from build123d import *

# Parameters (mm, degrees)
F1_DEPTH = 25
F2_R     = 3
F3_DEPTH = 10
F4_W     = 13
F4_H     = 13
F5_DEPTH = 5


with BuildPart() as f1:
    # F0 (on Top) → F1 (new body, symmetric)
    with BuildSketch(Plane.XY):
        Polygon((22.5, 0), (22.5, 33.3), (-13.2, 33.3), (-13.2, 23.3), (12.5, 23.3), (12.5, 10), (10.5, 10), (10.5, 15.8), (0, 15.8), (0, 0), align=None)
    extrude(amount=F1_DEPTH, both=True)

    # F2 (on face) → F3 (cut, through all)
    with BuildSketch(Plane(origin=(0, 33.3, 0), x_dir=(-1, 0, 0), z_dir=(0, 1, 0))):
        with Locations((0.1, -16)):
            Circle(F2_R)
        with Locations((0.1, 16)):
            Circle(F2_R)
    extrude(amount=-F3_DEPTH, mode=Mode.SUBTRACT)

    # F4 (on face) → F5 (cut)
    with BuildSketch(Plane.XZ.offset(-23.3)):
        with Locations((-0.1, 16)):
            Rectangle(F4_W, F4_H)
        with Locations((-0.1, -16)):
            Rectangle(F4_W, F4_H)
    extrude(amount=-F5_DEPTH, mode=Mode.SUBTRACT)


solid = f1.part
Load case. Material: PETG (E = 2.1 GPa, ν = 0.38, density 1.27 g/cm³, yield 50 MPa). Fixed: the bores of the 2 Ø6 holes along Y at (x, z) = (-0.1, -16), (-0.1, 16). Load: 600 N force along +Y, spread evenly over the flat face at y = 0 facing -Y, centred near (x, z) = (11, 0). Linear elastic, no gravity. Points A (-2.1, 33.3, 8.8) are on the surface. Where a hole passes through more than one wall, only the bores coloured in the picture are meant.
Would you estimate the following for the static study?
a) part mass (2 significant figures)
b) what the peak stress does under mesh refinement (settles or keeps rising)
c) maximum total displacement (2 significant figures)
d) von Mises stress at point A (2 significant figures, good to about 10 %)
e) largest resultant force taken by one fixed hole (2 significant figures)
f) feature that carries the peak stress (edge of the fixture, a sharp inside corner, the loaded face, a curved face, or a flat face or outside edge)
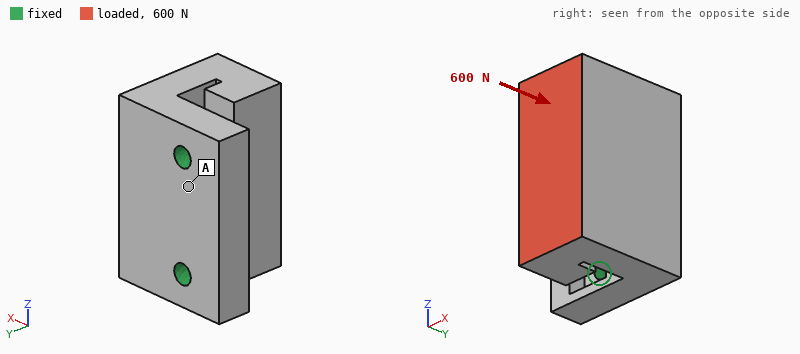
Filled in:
47 g
keeps rising
0.51 mm
3.8 MPa
300 N
edge of the fixture
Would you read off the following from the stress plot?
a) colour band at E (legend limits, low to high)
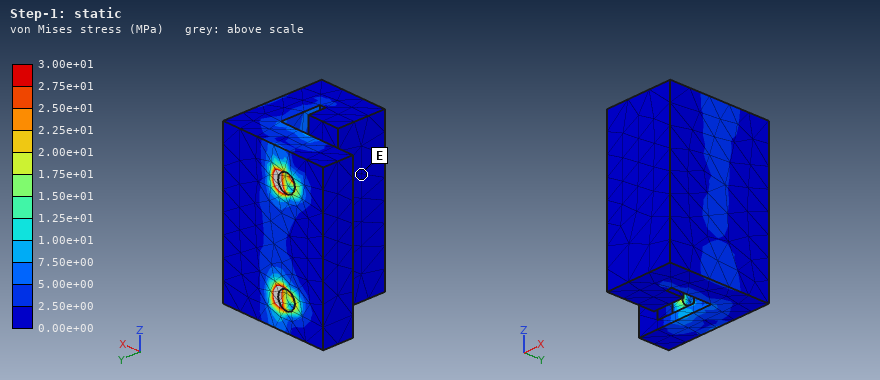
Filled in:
0.00e+00 to 2.50e+00 MPa
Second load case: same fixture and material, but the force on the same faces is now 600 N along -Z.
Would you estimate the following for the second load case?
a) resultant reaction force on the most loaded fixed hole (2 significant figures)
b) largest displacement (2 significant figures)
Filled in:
640 N
0.78 mm
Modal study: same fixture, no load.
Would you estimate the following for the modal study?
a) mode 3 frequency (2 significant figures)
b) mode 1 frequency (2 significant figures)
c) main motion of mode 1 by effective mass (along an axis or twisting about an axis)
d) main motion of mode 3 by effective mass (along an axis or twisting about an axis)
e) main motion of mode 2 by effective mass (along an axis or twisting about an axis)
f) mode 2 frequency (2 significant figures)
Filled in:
1700 Hz
600 Hz
along X
along Y
along Z
1100 Hz
